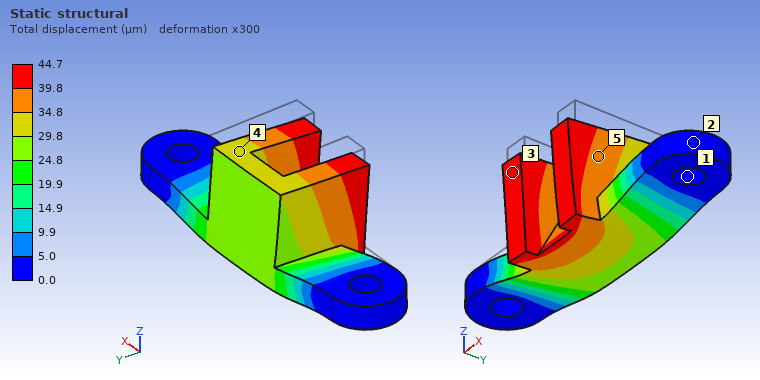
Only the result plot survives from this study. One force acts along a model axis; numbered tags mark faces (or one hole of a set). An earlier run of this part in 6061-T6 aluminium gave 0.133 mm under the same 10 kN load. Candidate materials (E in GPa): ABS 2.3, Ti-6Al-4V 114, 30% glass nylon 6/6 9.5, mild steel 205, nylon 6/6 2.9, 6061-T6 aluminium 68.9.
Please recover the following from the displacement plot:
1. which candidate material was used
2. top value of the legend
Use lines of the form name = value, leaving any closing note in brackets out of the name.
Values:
which candidate material was used = mild steel
top value of the legend = 44.7 µm
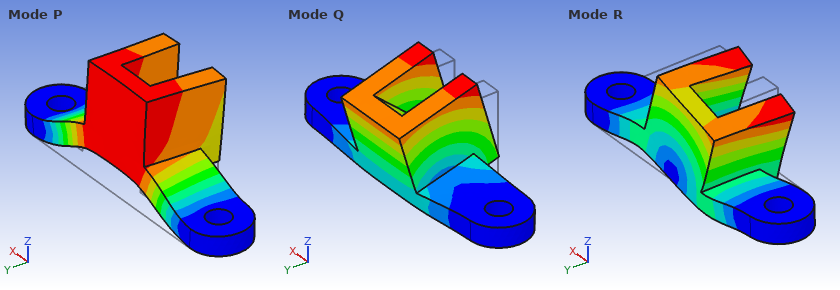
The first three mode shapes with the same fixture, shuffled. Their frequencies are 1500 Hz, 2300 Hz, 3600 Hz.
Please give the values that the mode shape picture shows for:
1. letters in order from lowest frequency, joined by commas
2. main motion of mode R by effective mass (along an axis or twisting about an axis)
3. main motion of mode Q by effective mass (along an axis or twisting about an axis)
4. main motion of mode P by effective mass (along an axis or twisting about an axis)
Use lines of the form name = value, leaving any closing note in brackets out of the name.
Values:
letters in order from lowest frequency, joined by commas = Q, P, R
main motion of mode R by effective mass = along X
main motion of mode Q by effective mass = along Y
main motion of mode P by effective mass = along Z
